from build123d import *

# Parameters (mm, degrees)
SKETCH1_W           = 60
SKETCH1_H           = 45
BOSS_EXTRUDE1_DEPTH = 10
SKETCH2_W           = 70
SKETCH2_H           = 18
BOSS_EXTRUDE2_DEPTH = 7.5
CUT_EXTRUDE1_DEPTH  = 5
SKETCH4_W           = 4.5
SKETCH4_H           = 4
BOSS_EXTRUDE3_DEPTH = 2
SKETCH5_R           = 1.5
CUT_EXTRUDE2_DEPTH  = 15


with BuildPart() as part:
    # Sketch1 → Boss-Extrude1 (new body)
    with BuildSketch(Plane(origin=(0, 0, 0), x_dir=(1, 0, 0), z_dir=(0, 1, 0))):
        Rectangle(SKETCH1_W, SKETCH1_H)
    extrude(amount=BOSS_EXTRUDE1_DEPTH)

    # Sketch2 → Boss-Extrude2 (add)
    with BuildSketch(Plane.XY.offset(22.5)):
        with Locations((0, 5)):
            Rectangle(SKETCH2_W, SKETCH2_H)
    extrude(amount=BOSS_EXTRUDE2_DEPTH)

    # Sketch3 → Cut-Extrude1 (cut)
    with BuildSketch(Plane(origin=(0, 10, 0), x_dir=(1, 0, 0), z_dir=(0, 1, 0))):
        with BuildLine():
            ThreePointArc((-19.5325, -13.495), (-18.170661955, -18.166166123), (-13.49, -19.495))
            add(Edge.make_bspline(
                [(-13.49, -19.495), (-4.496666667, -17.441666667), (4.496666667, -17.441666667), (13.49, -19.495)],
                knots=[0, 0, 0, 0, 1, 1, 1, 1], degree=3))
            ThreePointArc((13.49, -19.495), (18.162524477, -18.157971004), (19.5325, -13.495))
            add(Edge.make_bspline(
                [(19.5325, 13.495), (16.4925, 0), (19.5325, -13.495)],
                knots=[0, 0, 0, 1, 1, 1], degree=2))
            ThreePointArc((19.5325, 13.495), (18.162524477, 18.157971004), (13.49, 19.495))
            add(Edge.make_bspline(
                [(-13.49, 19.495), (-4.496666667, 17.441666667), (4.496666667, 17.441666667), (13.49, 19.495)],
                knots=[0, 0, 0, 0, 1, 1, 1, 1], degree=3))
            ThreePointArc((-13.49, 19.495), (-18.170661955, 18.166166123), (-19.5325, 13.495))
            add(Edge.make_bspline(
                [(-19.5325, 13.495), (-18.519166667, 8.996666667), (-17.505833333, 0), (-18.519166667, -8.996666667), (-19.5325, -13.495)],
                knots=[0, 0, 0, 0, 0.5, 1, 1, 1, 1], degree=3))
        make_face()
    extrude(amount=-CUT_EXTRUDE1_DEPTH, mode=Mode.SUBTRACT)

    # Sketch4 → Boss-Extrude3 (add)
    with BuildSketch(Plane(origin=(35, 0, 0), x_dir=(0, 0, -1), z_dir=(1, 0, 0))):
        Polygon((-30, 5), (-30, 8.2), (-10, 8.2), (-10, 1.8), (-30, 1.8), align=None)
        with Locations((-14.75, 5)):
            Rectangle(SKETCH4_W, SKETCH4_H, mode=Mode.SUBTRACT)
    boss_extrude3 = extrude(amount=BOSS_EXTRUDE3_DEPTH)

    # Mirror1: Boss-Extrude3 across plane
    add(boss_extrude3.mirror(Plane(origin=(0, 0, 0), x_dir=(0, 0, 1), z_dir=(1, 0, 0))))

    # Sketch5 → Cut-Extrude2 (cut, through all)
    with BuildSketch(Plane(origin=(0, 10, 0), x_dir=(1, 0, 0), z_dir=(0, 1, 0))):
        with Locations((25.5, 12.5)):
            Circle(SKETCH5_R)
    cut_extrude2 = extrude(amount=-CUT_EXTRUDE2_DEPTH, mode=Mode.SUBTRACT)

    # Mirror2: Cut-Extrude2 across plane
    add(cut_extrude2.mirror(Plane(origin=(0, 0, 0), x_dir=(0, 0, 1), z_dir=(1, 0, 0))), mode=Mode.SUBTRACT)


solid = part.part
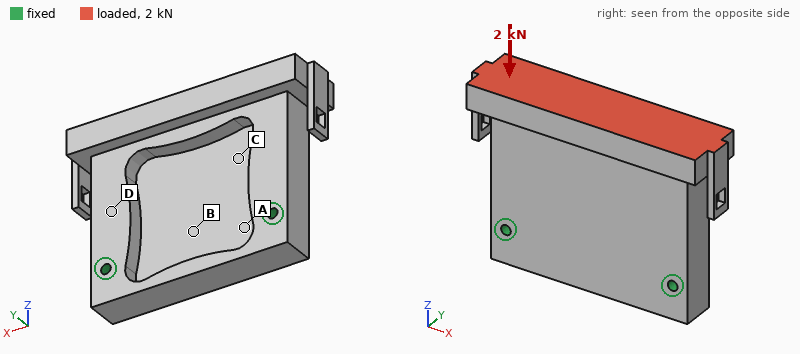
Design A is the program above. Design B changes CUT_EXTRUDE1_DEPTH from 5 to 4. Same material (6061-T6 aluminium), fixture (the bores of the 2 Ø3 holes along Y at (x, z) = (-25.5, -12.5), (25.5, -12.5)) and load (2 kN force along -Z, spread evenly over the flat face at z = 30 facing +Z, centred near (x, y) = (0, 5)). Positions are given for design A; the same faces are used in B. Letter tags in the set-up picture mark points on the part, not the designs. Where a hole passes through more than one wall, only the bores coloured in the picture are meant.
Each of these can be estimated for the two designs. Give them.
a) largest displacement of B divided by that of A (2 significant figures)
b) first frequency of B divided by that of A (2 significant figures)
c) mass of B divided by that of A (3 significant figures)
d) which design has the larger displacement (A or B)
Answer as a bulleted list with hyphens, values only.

- 0.81
- 1.0
- 1.05
- A
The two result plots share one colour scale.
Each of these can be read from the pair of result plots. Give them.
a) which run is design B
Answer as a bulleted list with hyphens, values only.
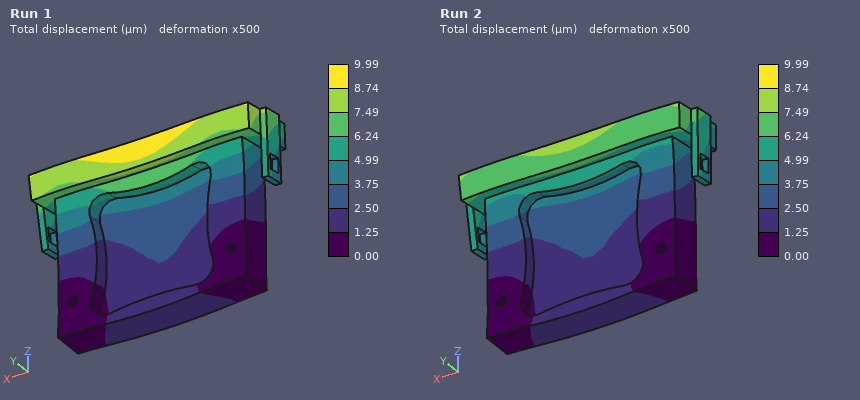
- Run 2
